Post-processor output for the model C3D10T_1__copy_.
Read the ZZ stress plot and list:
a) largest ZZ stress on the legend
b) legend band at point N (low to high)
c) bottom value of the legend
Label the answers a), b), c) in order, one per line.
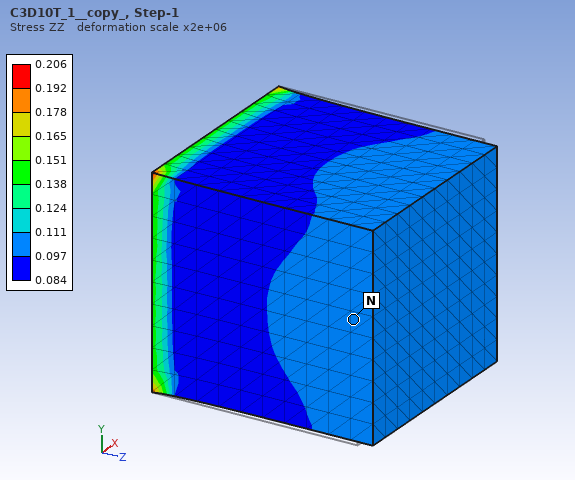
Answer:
a) 0.206
b) 0.097 to 0.111
c) 0.084
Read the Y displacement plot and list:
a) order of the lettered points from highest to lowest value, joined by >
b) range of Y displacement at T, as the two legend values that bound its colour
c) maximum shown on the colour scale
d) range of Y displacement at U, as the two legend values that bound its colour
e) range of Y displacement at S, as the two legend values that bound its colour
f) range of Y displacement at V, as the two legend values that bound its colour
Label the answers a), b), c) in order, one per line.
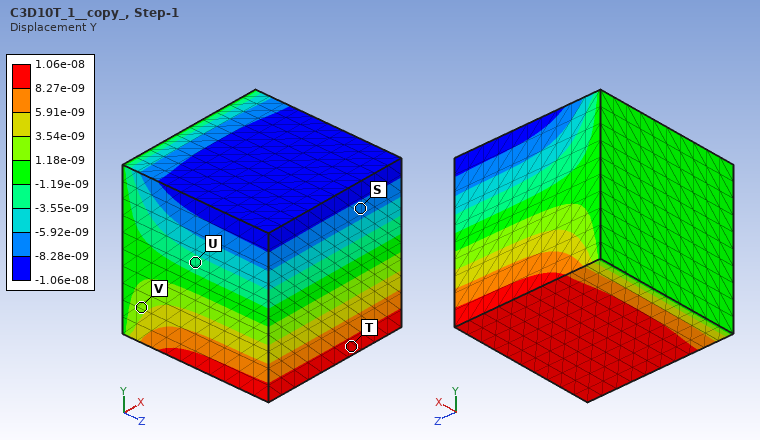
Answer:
a) T > V > U > S
b) 8.27e-09 to 1.06e-08
c) 1.06e-08
d) -3.55e-09 to -1.19e-09
e) -8.28e-09 to -5.92e-09
f) 1.18e-09 to 3.54e-09
